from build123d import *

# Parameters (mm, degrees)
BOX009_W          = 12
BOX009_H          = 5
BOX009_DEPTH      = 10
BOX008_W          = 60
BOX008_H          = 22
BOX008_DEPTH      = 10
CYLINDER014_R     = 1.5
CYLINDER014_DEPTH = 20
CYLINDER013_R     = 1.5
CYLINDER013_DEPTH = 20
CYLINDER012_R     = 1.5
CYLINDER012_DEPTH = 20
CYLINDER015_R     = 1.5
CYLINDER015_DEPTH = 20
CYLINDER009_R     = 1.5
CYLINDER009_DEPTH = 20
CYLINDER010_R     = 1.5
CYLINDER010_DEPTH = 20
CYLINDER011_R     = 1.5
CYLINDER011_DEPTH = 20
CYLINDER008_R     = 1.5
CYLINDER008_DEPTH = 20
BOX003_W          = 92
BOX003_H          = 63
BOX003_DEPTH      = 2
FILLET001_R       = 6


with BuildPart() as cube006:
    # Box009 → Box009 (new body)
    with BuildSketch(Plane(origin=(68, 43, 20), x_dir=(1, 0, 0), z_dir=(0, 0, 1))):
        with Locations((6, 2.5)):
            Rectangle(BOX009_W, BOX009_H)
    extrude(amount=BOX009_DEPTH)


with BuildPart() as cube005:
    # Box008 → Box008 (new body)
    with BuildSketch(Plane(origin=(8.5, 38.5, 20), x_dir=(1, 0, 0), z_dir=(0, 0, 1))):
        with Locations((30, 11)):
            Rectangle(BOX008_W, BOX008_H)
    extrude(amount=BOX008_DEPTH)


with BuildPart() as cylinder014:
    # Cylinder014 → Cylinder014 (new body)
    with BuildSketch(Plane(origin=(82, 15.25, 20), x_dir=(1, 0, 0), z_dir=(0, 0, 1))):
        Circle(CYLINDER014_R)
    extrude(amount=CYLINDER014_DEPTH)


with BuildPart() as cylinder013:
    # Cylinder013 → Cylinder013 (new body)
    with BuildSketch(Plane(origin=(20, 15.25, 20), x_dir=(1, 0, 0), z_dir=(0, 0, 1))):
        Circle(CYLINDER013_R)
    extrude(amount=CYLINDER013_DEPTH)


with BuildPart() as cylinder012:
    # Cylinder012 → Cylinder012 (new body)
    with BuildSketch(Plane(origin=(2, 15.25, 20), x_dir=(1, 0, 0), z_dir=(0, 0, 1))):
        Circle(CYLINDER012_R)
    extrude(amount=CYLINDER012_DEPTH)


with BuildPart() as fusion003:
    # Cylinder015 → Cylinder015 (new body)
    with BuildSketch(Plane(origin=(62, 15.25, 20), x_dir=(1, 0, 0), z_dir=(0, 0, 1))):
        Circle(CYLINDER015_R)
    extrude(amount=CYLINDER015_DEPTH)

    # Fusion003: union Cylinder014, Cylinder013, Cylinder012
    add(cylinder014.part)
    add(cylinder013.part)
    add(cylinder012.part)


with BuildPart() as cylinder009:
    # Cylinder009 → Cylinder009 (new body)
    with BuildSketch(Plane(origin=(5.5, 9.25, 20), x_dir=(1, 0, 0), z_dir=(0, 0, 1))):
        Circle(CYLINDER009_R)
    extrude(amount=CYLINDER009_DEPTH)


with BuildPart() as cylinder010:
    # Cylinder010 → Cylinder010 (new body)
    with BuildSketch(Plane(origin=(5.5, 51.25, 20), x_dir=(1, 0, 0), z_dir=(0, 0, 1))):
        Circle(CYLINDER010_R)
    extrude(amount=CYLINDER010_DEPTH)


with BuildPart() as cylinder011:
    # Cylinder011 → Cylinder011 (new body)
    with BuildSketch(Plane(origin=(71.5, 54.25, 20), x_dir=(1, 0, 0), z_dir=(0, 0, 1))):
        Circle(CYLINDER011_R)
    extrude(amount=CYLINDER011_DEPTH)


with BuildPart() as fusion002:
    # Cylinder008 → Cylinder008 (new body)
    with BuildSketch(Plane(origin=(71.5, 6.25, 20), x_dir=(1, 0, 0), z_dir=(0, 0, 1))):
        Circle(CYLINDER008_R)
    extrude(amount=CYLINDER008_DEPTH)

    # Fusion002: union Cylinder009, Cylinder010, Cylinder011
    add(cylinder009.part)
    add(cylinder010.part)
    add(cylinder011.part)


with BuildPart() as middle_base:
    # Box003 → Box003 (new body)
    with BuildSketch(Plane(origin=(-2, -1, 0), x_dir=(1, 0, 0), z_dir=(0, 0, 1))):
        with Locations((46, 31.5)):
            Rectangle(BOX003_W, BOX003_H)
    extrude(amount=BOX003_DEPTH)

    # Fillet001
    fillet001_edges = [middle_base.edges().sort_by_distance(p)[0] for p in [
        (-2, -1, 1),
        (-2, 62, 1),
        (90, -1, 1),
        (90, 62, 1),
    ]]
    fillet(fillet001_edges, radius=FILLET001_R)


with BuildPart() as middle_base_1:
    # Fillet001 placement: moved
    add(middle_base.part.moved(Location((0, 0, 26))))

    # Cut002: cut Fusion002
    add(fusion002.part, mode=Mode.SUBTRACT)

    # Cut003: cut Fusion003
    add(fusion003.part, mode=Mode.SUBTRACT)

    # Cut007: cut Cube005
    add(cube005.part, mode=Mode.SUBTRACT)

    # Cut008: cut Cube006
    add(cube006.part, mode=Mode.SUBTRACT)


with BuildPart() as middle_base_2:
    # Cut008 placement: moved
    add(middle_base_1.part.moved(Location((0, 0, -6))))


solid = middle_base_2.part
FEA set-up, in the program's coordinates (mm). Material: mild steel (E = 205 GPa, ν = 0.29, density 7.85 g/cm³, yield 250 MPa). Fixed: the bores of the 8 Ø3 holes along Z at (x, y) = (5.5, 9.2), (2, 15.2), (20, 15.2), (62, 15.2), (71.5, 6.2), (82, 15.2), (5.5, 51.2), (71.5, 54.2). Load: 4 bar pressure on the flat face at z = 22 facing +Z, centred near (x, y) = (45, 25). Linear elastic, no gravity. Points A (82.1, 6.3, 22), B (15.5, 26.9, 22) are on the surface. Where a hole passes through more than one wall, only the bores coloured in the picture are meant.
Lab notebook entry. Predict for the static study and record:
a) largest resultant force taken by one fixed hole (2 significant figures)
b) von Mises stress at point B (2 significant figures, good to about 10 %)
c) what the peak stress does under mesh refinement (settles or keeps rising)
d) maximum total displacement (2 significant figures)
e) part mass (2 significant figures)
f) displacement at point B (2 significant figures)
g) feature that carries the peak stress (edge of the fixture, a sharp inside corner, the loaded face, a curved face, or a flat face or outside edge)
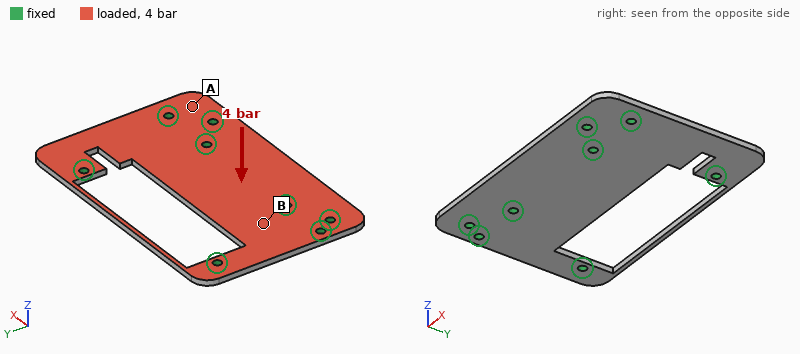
480 N
53 MPa
keeps rising
0.14 mm
68 g
0.021 mm
edge of the fixture
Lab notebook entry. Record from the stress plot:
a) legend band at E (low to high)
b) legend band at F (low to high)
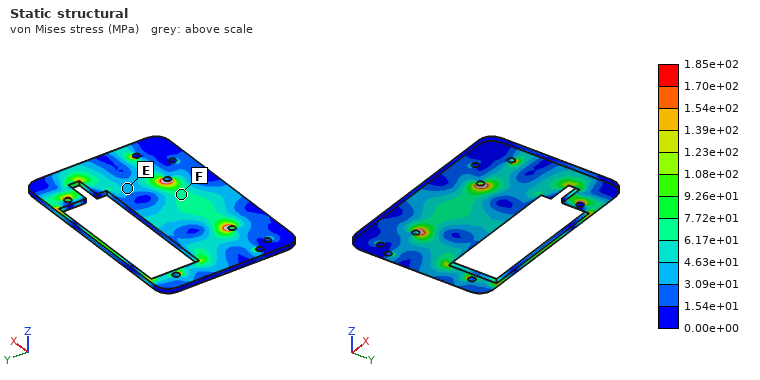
3.09e+01 to 4.63e+01 MPa
6.17e+01 to 7.72e+01 MPa
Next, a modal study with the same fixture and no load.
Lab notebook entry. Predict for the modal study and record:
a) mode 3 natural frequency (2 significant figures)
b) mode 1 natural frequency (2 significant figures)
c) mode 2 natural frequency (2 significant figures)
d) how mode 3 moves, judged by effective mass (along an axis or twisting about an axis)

3100 Hz
2100 Hz
2400 Hz
along Z
